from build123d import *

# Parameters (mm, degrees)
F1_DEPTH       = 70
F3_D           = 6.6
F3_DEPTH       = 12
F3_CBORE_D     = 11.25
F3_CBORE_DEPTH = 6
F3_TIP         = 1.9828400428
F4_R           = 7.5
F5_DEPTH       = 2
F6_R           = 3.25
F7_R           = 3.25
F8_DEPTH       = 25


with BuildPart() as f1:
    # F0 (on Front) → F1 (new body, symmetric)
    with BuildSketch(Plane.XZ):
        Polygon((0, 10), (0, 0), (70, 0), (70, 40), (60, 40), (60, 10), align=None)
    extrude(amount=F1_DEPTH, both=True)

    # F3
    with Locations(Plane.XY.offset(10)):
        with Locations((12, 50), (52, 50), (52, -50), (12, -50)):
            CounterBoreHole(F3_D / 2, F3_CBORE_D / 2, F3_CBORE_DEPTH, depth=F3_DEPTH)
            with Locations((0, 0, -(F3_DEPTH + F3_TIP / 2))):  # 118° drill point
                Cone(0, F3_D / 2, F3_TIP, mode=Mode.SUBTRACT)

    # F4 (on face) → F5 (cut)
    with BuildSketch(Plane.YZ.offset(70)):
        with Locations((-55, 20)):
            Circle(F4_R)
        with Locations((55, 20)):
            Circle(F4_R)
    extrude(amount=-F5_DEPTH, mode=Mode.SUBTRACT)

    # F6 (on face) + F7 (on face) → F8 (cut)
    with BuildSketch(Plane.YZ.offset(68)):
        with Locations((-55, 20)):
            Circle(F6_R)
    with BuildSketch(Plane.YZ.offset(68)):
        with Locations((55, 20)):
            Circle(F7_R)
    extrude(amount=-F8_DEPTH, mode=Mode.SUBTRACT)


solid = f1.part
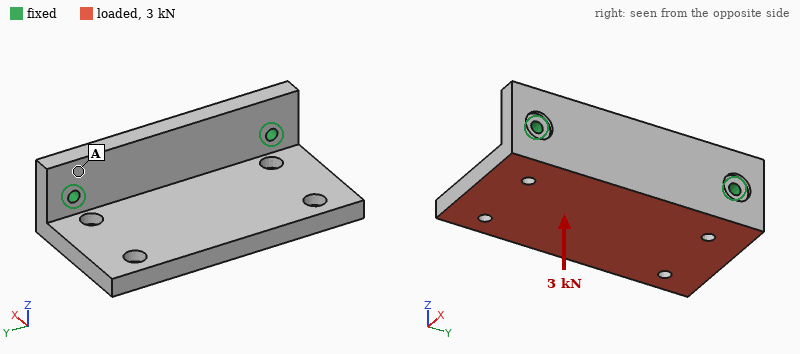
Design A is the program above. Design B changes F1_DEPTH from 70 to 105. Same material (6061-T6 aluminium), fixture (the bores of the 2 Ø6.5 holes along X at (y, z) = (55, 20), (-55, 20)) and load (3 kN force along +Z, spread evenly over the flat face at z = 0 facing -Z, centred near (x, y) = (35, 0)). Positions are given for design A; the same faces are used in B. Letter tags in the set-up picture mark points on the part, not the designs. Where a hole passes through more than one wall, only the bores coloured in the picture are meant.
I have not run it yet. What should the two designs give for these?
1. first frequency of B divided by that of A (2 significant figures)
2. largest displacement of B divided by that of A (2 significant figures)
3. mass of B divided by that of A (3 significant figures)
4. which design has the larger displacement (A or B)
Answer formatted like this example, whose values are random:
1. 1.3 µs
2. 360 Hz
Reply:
1. 0.93
2. 0.73
3. 1.52
4. A
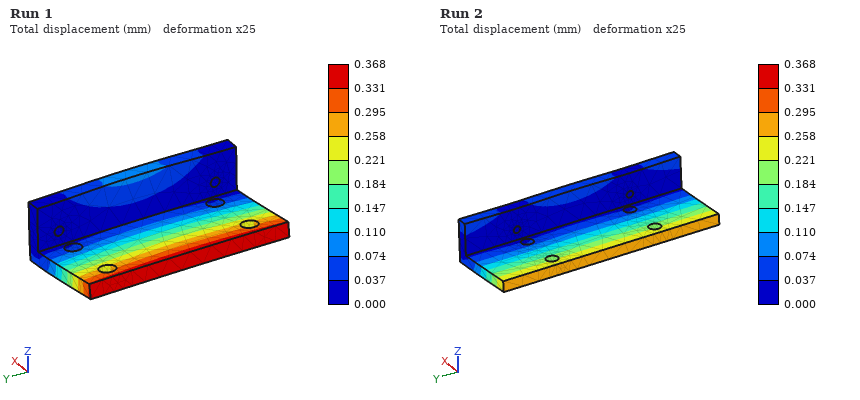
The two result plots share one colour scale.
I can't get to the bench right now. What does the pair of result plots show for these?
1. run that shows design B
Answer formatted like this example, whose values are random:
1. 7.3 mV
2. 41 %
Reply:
1. Run 2
